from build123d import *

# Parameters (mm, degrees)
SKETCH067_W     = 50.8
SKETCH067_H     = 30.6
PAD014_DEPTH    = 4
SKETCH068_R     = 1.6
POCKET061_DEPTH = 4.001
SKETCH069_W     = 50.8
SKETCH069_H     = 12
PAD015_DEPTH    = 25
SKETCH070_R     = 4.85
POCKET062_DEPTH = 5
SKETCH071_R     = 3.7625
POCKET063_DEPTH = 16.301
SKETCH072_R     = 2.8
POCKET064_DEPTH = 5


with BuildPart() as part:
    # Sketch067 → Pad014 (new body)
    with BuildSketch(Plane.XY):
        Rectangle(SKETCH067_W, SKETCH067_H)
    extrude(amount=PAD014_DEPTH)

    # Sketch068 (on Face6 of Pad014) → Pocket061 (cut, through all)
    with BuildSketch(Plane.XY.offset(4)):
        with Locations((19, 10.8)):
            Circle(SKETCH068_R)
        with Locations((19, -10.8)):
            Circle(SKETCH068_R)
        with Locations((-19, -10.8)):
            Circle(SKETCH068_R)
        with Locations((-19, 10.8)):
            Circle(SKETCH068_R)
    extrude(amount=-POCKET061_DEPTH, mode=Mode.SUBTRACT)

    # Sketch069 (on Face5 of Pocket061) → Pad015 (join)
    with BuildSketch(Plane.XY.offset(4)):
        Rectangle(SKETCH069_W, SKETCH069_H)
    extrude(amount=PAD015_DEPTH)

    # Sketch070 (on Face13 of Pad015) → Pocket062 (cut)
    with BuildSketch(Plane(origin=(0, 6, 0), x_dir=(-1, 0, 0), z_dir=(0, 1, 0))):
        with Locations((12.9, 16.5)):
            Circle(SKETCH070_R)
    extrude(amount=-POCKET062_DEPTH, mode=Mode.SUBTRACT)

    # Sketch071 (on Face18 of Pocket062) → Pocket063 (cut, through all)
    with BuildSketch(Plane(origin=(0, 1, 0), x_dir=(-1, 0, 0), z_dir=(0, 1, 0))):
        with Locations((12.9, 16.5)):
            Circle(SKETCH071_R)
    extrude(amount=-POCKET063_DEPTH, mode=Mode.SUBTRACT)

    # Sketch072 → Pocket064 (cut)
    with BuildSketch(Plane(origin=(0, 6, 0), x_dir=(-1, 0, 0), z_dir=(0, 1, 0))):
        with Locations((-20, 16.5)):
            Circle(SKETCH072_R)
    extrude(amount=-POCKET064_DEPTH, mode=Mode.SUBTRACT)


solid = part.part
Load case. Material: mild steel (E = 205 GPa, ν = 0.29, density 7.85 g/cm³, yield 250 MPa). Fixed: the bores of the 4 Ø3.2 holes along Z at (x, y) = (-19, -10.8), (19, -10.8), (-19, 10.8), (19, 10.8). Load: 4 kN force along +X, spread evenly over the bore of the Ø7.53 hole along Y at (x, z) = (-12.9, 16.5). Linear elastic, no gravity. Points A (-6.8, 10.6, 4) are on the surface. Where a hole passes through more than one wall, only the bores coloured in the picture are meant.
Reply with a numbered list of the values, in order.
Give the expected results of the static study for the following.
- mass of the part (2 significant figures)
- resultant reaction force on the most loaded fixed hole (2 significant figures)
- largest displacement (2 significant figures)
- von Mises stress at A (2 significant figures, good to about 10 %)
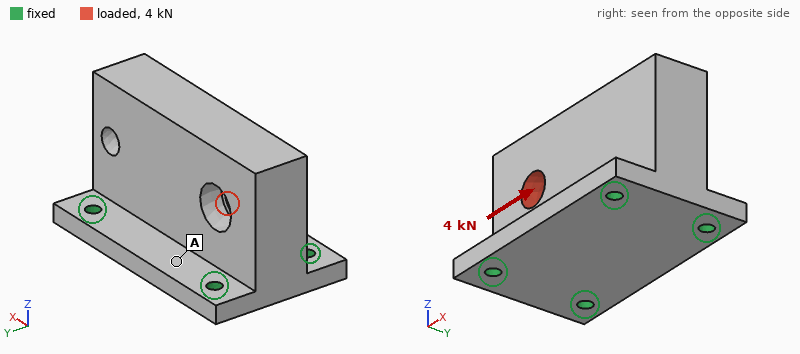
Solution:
1. 160 g
2. 1.4 kN
3. 8.8 µm
4. 16 MPa
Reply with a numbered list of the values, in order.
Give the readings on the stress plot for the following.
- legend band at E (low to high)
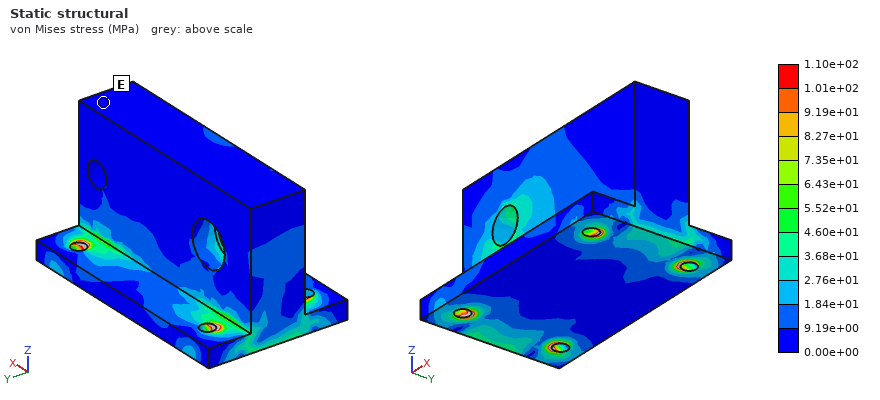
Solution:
1. 0.00e+00 to 9.19e+00 MPa
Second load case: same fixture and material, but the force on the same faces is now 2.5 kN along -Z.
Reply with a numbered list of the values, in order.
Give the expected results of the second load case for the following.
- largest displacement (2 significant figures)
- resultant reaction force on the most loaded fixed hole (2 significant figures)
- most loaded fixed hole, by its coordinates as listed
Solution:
1. 6.8 µm
2. 1.3 kN
3. (-19, -10.8)
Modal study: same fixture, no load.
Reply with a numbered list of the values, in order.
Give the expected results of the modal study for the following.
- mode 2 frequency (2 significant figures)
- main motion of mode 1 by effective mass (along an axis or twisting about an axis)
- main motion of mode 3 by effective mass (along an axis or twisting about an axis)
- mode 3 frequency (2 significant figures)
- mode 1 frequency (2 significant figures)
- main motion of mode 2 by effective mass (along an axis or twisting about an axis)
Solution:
1. 12 kHz
2. along Y
3. along Z
4. 13 kHz
5. 6900 Hz
6. along X
